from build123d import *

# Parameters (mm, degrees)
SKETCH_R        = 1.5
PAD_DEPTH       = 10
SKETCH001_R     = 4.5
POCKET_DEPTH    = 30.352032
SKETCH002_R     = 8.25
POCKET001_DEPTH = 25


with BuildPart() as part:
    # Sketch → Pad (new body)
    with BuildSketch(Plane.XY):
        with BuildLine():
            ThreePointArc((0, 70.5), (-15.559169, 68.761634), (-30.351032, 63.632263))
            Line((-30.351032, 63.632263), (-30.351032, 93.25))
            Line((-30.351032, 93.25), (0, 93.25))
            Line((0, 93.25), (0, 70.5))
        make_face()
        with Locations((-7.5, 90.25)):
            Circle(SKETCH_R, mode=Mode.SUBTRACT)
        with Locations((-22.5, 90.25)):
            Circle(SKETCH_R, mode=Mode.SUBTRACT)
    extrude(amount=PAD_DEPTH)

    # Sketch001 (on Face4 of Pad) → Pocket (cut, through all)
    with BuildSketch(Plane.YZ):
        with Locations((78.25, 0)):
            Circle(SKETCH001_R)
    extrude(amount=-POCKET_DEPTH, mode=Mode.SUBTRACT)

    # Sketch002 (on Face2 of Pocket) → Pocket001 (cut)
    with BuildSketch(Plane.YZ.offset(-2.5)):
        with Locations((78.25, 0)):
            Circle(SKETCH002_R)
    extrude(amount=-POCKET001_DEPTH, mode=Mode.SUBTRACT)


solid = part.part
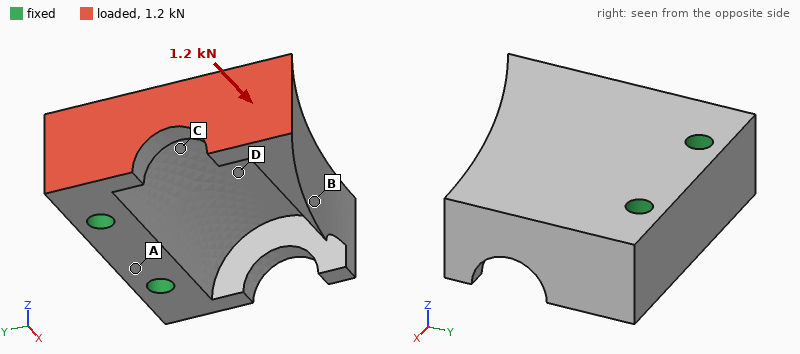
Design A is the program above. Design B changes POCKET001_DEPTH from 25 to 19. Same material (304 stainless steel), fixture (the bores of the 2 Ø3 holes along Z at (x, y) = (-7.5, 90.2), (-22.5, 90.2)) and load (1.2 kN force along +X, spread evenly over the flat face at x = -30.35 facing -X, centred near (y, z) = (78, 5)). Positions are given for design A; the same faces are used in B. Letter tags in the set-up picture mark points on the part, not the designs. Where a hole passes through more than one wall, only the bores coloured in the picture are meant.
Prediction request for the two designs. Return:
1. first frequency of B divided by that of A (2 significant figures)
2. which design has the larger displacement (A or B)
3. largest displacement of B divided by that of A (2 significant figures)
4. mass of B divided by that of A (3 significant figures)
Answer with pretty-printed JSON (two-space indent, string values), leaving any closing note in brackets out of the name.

{
  "first frequency of B divided by that of A": "1.3",
  "which design has the larger displacement": "A",
  "largest displacement of B divided by that of A": "0.78",
  "mass of B divided by that of A": "1.10"
}
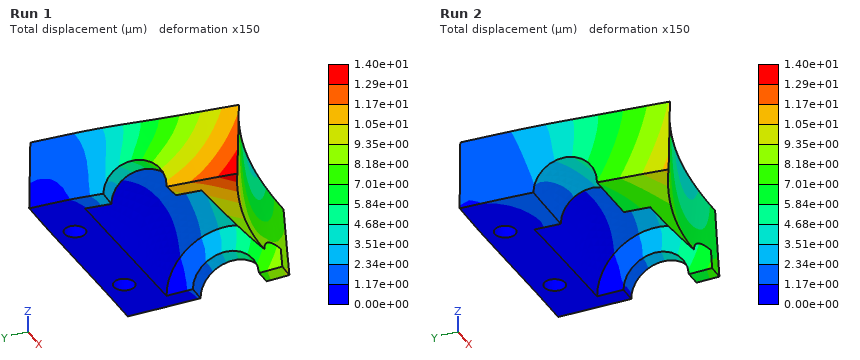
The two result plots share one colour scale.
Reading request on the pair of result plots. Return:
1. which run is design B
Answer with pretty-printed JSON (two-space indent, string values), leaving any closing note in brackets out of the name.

{
  "which run is design B": "Run 2"
}
